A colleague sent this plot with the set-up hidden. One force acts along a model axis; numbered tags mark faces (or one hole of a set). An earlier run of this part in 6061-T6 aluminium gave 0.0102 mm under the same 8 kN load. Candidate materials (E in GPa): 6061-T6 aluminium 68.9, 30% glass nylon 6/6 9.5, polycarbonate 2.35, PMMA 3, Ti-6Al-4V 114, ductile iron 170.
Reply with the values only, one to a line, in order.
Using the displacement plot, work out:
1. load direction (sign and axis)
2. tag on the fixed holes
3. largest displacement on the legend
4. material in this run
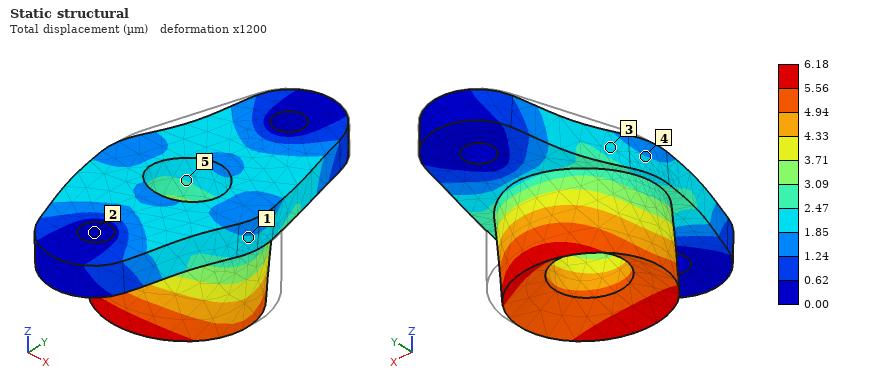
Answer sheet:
-Y
2
6.18 µm
Ti-6Al-4V
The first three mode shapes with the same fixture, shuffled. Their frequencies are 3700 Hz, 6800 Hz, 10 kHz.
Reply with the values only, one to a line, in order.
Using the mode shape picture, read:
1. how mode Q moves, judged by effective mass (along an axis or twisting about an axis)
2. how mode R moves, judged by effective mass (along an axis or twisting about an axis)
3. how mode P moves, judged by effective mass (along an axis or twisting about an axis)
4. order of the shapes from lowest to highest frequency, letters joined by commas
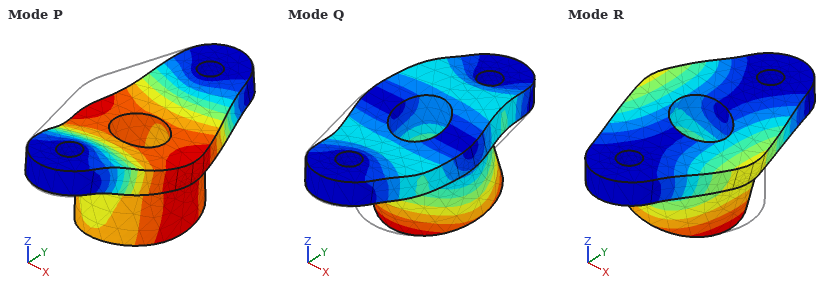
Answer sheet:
along Y
along X
along Z
R, P, Q
